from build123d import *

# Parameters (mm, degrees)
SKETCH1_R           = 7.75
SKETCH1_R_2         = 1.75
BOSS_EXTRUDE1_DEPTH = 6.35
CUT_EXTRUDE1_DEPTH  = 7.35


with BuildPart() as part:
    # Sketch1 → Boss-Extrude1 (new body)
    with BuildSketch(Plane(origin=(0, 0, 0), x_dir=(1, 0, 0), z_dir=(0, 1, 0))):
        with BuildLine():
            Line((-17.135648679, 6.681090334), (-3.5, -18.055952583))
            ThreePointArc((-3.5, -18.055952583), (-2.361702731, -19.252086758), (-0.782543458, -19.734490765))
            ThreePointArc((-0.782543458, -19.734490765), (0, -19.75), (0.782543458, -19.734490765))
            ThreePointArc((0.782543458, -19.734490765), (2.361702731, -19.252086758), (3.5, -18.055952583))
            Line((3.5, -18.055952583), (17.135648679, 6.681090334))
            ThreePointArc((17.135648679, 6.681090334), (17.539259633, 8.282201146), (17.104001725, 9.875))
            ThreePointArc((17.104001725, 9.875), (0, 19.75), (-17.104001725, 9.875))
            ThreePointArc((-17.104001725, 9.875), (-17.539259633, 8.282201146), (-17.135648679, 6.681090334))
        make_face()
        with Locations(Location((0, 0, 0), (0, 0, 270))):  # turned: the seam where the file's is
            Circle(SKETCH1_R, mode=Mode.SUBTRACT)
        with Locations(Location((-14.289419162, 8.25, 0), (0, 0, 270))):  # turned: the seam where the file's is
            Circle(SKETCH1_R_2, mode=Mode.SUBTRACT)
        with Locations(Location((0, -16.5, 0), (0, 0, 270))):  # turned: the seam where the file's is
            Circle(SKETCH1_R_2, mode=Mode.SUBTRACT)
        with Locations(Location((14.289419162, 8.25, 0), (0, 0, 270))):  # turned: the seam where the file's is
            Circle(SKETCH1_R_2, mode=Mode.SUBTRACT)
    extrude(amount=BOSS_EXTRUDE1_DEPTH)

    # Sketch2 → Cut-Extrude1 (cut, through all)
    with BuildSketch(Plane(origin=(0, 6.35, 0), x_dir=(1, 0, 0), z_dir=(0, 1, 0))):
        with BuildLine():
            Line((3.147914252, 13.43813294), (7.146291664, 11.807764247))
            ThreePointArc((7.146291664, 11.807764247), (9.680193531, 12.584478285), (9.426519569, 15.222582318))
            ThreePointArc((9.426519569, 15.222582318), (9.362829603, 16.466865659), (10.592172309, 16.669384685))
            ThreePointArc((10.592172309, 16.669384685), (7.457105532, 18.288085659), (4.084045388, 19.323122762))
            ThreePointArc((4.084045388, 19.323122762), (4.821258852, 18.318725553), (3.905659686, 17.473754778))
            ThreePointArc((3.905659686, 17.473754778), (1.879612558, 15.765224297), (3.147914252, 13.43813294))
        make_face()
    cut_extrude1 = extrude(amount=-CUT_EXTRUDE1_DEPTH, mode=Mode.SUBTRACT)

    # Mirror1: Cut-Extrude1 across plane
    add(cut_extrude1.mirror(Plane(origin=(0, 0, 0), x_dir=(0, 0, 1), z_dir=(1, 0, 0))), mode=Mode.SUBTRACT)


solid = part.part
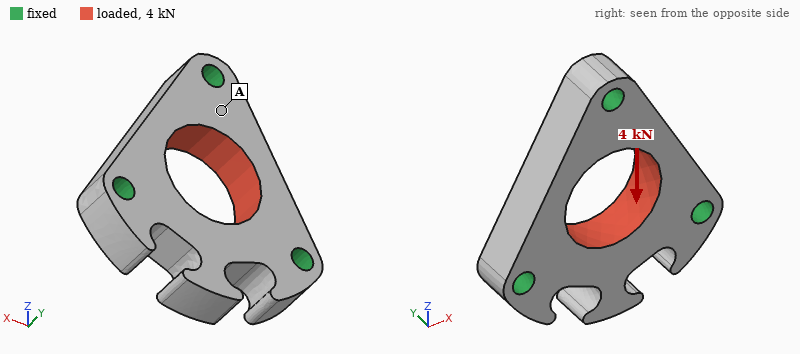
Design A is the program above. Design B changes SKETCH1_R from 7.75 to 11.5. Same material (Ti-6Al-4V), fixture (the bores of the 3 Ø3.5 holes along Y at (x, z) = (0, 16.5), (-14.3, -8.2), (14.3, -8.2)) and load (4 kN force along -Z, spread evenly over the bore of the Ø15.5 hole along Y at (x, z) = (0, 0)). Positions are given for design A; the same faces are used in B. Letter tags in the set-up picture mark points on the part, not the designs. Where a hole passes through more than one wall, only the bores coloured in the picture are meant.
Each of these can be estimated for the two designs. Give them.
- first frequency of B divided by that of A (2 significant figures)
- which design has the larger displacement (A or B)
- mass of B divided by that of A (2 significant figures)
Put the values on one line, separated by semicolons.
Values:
0.68; B; 0.60
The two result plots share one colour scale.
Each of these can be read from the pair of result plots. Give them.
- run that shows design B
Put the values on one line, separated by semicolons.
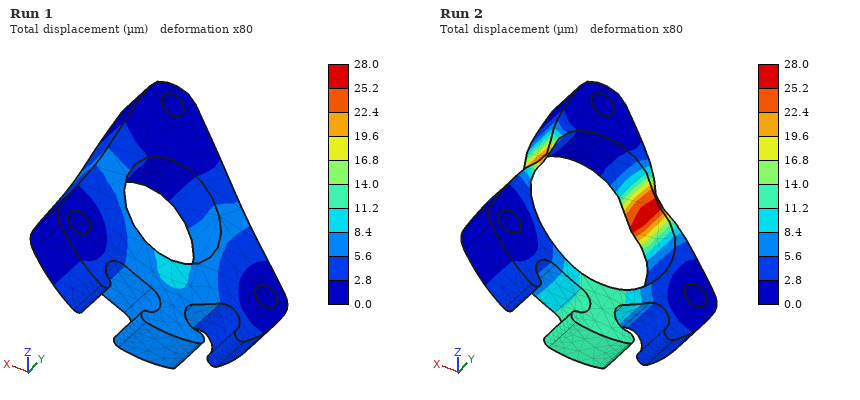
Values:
Run 2
